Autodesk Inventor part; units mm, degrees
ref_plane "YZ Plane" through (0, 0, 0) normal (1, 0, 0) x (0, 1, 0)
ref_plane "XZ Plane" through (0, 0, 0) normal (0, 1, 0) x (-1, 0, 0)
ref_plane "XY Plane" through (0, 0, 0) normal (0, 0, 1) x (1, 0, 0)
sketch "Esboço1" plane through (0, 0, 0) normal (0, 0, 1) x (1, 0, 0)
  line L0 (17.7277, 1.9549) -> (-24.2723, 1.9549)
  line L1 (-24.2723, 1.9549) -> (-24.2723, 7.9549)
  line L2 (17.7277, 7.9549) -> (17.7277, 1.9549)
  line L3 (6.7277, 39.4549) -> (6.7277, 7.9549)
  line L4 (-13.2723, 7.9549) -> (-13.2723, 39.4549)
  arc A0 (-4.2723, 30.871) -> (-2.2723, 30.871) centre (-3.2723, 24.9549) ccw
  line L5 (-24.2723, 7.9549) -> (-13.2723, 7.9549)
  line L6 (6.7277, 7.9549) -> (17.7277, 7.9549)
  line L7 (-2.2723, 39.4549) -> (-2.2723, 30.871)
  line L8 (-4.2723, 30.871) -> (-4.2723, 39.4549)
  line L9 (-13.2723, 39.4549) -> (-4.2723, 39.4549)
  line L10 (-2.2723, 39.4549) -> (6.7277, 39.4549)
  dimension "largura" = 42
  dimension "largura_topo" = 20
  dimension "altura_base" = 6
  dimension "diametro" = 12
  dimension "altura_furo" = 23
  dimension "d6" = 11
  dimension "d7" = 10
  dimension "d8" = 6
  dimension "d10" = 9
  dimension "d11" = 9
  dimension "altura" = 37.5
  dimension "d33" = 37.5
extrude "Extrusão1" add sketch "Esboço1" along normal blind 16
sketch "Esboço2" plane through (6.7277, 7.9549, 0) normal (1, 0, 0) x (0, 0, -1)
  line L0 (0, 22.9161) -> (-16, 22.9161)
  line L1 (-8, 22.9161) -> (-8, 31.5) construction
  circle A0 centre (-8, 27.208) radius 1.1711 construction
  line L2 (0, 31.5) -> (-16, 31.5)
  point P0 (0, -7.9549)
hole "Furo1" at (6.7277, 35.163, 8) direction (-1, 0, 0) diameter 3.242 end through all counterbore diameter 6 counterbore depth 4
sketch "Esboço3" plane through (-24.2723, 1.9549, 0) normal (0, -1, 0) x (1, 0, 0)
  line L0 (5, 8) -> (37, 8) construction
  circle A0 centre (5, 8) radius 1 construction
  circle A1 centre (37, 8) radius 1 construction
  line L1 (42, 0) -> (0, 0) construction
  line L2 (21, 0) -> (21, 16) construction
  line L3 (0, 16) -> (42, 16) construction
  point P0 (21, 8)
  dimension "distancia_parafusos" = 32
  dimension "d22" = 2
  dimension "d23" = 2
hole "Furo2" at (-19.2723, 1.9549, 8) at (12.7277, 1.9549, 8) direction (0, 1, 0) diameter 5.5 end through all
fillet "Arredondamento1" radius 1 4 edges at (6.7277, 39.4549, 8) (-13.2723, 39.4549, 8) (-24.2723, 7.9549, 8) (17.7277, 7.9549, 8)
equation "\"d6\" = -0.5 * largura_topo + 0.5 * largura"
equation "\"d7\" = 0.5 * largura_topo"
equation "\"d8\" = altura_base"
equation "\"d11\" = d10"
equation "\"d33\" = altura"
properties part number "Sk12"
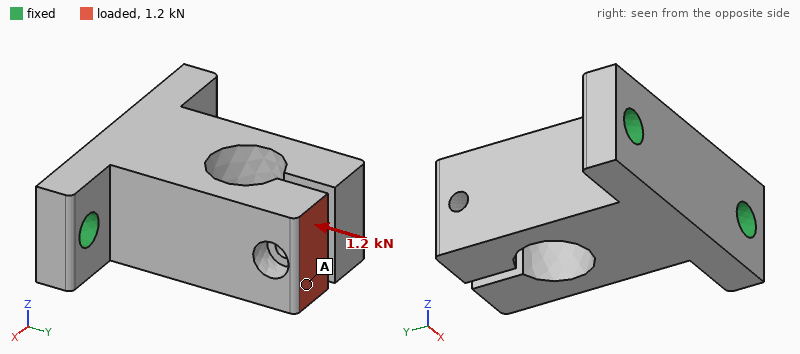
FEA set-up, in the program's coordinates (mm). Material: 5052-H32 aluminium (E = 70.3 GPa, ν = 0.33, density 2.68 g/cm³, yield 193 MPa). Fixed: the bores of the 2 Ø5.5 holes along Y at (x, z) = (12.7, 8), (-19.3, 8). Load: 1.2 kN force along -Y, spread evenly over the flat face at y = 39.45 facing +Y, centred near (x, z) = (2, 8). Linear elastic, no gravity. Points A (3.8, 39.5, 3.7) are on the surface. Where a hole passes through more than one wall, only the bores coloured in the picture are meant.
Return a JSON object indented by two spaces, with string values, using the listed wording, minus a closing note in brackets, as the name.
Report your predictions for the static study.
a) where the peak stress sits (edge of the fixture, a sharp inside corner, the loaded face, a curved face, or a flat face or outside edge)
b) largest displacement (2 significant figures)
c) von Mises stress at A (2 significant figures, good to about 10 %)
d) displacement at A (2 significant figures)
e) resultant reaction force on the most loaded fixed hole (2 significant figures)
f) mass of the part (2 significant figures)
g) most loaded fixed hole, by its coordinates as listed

{
  "where the peak stress sits": "a curved face",
  "largest displacement": "71 µm",
  "von Mises stress at A": "12 MPa",
  "displacement at A": "61 µm",
  "resultant reaction force on the most loaded fixed hole": "870 N",
  "mass of the part": "31 g",
  "most loaded fixed hole, by its coordinates as listed": "(12.7, 8)"
}
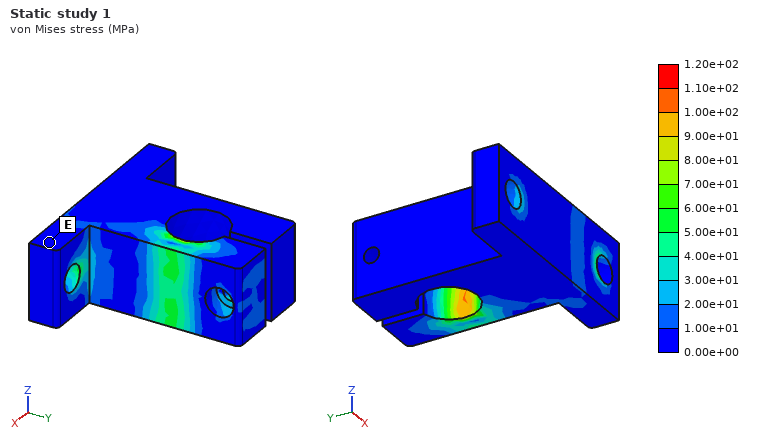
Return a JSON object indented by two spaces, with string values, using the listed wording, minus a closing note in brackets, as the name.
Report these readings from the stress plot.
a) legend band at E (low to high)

{
  "legend band at E": "0.00e+00 to 1.00e+01 MPa"
}
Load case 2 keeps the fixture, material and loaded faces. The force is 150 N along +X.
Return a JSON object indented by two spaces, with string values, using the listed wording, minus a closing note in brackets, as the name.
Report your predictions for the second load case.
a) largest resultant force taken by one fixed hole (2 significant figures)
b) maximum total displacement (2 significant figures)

{
  "largest resultant force taken by one fixed hole": "240 N",
  "maximum total displacement": "60 µm"
}
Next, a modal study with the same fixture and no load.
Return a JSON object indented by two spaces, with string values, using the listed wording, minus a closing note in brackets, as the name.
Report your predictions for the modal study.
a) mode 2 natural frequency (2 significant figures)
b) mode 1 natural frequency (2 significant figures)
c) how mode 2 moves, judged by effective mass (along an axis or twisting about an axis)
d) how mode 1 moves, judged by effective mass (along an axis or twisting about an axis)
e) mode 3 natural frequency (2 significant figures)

{
  "mode 2 natural frequency": "5500 Hz",
  "mode 1 natural frequency": "4500 Hz",
  "how mode 2 moves, judged by effective mass": "along X",
  "how mode 1 moves, judged by effective mass": "along Z",
  "mode 3 natural frequency": "6100 Hz"
}
